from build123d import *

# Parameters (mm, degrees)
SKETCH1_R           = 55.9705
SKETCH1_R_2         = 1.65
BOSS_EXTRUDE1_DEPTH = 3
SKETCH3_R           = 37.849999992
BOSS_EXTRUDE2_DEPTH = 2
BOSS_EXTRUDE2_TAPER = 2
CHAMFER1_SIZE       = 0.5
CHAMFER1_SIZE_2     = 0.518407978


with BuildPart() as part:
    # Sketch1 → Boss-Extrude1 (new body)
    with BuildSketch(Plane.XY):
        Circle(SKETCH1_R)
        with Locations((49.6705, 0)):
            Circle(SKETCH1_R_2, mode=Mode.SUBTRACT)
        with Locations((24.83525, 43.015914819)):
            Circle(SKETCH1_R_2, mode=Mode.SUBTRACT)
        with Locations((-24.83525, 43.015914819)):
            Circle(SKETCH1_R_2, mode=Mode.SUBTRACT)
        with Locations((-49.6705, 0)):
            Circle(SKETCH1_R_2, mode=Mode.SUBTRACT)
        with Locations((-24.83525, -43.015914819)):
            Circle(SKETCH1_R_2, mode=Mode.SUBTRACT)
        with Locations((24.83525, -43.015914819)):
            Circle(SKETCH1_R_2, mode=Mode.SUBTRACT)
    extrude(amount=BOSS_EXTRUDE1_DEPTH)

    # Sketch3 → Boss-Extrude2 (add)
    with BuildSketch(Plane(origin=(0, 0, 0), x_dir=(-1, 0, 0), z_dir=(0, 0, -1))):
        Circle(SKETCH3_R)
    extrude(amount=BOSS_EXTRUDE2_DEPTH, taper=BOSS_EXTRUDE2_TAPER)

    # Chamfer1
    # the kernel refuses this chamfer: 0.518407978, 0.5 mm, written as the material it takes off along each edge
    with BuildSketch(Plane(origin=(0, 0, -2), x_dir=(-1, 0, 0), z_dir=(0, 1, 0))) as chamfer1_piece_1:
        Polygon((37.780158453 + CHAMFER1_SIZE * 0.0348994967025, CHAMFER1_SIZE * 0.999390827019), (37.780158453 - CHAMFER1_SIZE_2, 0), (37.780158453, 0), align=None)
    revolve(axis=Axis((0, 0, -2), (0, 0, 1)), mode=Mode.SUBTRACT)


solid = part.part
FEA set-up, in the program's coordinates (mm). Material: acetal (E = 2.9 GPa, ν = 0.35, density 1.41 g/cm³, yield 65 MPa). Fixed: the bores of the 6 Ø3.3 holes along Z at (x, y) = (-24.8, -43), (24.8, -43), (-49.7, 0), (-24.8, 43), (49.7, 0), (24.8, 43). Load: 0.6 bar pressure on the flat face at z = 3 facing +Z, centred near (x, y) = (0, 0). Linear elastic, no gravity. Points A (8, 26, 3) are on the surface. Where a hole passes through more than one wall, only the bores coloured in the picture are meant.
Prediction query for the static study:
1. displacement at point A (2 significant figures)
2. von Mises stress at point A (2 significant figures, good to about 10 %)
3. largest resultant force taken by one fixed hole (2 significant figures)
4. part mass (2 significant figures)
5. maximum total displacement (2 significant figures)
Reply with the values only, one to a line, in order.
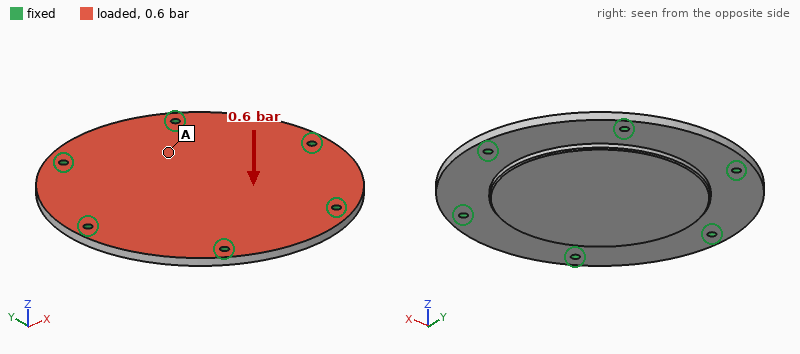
0.30 mm
2.7 MPa
120 N
54 g
0.44 mm
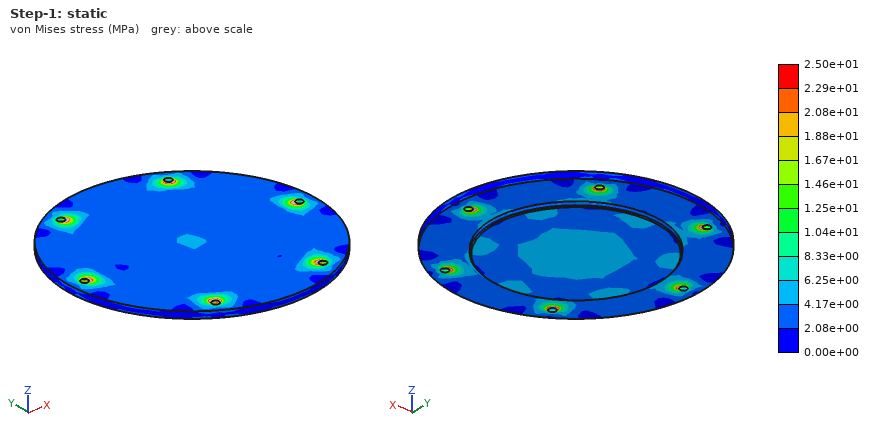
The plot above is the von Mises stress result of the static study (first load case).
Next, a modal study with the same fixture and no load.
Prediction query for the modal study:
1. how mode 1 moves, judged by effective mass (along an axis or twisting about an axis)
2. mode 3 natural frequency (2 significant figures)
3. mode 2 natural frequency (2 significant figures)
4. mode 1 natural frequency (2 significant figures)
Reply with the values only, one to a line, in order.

along Z
1600 Hz
1600 Hz
860 Hz
